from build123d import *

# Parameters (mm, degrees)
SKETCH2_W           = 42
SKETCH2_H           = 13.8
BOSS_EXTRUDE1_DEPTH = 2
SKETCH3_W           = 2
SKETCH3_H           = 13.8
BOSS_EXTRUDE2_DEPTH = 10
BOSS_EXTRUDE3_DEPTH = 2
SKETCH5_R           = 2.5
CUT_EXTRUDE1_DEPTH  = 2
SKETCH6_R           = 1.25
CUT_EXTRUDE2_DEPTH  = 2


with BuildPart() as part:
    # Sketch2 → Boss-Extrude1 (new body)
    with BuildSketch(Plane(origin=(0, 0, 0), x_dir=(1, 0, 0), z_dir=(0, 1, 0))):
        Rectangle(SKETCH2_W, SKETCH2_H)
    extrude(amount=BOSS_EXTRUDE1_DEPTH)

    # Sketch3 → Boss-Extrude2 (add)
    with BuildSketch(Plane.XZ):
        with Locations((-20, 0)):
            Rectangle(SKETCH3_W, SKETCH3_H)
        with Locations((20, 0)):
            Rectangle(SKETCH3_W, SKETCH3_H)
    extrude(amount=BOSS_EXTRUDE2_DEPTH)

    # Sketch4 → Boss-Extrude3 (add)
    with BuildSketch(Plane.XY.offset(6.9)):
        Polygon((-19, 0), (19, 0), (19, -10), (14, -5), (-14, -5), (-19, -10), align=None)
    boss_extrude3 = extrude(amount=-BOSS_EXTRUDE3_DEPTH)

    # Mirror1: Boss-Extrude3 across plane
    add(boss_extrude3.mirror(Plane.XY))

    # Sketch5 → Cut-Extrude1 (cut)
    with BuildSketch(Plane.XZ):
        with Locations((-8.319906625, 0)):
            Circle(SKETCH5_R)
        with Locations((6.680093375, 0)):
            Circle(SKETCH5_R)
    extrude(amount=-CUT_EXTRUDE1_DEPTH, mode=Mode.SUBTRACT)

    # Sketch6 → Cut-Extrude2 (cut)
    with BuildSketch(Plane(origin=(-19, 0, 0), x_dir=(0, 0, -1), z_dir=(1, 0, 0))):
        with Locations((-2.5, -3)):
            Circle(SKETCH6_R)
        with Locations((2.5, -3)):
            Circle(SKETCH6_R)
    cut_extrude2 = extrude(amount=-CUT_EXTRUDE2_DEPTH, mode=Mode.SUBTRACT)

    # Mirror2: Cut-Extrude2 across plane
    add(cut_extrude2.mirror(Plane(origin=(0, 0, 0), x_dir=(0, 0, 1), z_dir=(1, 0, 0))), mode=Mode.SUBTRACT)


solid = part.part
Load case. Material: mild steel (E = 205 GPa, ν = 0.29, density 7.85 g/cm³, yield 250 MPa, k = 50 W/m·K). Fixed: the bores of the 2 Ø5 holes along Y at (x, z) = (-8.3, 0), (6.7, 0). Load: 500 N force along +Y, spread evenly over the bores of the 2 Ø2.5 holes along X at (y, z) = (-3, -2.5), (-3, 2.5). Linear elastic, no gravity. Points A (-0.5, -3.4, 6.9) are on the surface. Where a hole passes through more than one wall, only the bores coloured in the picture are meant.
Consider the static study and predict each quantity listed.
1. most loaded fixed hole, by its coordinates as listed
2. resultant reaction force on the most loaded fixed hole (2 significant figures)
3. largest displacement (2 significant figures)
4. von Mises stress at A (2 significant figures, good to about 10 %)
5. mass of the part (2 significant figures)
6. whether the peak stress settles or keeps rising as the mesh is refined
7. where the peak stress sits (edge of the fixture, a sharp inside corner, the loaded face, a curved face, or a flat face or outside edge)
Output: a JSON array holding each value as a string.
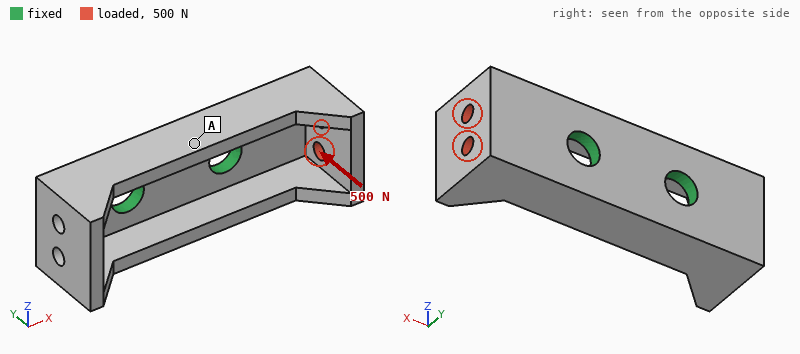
["(6.7, 0)", "860 N", "32 µm", "31 MPa", "19 g", "keeps rising", "edge of the fixture"]
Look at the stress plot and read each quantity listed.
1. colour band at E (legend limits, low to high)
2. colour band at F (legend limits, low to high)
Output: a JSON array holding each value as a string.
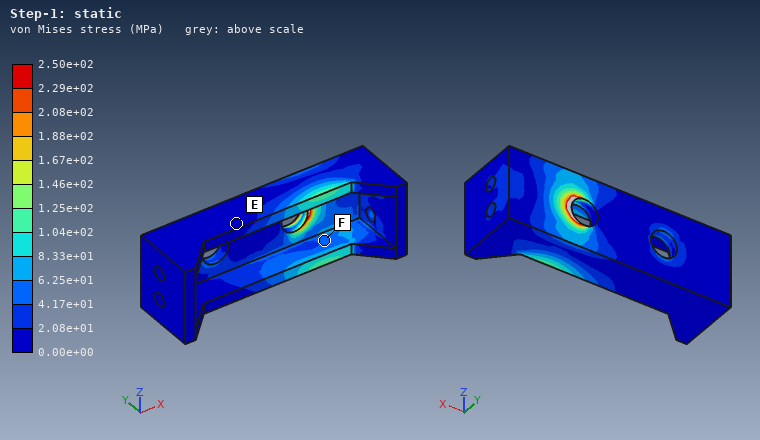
["0.00e+00 to 2.08e+01 MPa", "4.17e+01 to 6.25e+01 MPa"]
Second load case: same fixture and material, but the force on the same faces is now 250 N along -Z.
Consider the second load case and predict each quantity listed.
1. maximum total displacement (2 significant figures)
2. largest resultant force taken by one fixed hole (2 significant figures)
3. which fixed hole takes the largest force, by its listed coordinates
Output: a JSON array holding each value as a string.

["20 µm", "340 N", "(6.7, 0)"]
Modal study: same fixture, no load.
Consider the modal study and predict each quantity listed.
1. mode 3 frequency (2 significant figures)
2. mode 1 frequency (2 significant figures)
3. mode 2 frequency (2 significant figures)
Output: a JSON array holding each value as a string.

["10 kHz", "9100 Hz", "10 kHz"]
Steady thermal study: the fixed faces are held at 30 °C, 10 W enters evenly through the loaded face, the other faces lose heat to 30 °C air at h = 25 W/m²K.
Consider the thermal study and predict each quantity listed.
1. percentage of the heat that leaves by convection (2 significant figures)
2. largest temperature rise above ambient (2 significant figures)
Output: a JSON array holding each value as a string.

["11 %", "71 K"]
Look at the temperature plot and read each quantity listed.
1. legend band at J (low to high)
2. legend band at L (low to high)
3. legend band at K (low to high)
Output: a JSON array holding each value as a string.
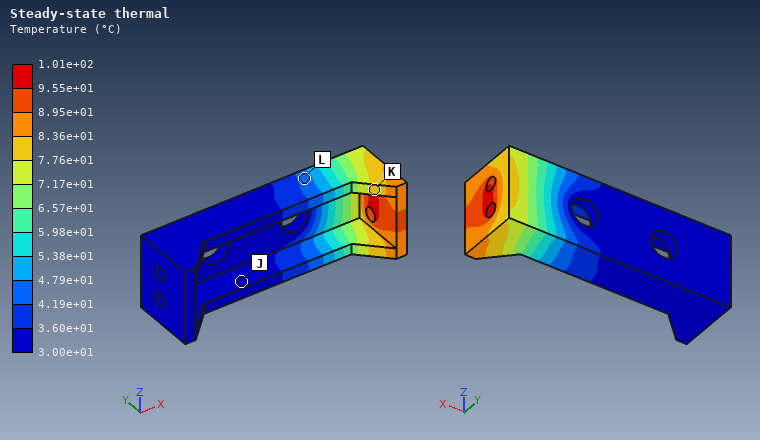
["3.00e+01 to 3.60e+01 °C", "4.19e+01 to 4.79e+01 °C", "7.76e+01 to 8.36e+01 °C"]
